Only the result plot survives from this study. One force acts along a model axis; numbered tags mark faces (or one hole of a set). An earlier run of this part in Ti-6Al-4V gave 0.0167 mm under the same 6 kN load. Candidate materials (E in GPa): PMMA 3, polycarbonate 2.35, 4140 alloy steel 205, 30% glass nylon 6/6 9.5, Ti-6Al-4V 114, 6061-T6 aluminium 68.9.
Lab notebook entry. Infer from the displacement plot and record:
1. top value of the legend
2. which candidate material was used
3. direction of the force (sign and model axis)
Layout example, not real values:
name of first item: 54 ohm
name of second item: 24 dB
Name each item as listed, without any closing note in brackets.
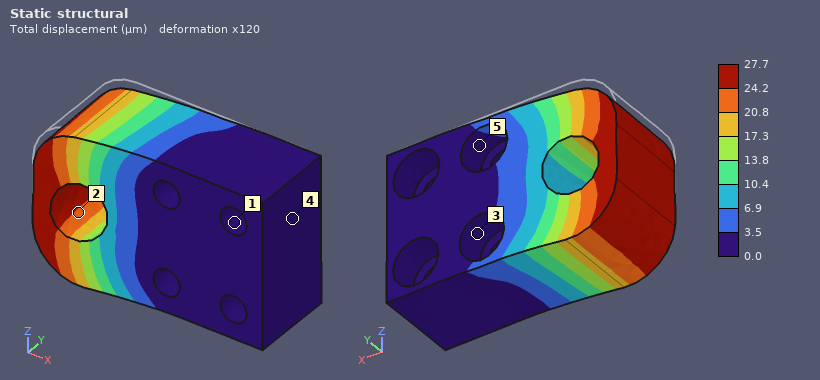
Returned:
top value of the legend: 27.7 µm
which candidate material was used: 6061-T6 aluminium
direction of the force: -Z
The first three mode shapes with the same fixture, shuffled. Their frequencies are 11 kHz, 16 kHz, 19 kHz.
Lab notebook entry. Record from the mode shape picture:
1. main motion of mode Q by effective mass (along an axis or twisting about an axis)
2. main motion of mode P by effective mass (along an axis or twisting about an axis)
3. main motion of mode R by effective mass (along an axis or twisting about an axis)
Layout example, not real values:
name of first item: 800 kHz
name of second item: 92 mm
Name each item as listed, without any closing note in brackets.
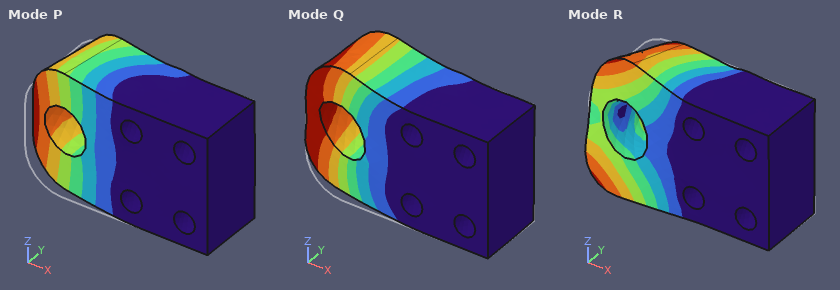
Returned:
main motion of mode Q by effective mass: along Z
main motion of mode P by effective mass: along Y
main motion of mode R by effective mass: twisting about X
